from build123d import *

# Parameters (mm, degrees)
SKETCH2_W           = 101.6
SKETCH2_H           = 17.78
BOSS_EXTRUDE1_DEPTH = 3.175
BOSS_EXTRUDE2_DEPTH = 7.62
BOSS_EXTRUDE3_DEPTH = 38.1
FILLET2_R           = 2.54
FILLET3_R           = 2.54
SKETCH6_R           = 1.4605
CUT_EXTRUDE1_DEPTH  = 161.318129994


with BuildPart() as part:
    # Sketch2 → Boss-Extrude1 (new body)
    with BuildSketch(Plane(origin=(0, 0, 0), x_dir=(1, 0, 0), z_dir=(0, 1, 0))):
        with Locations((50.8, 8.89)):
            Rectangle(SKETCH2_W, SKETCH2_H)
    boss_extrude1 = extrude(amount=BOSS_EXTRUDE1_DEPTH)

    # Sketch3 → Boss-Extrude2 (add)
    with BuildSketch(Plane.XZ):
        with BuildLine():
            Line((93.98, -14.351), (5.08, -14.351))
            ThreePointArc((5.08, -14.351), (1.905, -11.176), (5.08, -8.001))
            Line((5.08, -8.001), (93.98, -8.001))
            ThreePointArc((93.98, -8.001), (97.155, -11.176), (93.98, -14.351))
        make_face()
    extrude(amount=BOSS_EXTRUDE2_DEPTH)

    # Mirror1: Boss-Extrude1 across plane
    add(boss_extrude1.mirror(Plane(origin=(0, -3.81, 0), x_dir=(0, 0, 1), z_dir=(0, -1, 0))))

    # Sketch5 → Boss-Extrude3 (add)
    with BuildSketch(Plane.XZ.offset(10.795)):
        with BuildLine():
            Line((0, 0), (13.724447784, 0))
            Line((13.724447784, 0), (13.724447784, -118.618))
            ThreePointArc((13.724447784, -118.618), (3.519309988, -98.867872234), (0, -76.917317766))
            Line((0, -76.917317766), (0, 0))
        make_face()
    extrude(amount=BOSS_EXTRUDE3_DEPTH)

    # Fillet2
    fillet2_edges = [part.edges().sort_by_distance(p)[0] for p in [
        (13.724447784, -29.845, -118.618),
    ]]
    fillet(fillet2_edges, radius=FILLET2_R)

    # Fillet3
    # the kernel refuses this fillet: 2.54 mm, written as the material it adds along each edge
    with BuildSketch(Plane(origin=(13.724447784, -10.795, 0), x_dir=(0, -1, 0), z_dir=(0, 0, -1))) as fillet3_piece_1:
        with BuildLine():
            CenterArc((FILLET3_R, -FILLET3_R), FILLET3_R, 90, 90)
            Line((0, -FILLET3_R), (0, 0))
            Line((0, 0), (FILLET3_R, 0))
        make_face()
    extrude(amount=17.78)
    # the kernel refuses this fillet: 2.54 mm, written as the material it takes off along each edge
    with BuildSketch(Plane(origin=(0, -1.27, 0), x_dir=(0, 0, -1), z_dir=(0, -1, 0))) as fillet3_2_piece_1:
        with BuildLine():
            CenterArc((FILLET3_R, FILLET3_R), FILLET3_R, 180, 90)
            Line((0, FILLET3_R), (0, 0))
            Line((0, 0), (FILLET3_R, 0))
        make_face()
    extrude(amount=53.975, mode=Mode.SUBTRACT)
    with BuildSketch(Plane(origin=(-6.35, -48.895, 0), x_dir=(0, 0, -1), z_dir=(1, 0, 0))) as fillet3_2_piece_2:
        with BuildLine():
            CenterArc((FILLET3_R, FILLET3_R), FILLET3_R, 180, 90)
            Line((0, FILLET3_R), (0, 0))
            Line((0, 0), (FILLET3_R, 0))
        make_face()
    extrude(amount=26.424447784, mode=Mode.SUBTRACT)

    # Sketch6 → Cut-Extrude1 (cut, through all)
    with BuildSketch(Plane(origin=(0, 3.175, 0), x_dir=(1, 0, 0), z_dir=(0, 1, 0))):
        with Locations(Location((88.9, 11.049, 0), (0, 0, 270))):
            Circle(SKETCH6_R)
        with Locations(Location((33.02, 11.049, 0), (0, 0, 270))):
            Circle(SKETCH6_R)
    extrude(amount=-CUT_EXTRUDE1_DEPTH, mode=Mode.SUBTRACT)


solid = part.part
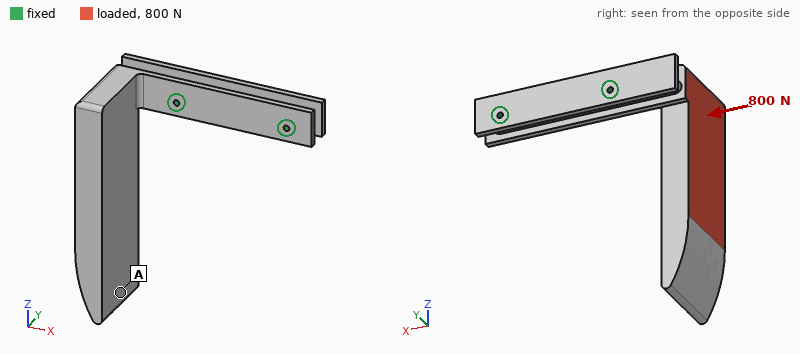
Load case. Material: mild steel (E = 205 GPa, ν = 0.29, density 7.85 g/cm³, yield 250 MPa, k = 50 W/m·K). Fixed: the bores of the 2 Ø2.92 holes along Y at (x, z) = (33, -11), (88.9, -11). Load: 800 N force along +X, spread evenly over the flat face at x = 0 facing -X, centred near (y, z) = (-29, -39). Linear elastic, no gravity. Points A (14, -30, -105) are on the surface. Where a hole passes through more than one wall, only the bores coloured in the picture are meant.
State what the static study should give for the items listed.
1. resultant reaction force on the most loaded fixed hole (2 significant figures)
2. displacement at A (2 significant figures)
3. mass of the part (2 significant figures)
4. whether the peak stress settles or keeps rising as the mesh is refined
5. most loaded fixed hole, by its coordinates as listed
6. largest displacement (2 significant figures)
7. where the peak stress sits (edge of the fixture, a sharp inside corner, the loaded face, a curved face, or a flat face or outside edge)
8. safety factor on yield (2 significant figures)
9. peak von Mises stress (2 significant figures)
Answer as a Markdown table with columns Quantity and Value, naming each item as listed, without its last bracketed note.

| Quantity | Value |
|---|---|
| resultant reaction force on the most loaded fixed hole | 1.2 kN |
| displacement at A | 0.22 mm |
| mass of the part | 550 g |
| whether the peak stress settles or keeps rising as the mesh is refined | settles |
| most loaded fixed hole, by its coordinates as listed | (33, -11) |
| largest displacement | 0.26 mm |
| where the peak stress sits | a curved face |
| safety factor on yield | 0.77 |
| peak von Mises stress | 320 MPa |
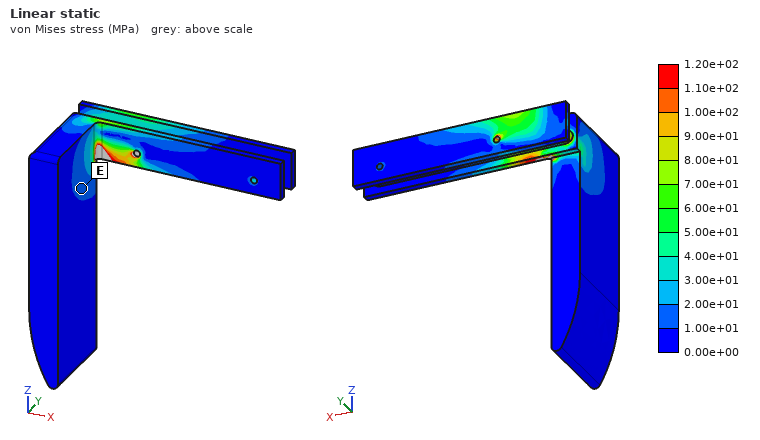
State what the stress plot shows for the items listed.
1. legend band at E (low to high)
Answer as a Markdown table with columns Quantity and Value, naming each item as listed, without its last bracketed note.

| Quantity | Value |
|---|---|
| legend band at E | 1.00e+01 to 2.00e+01 MPa |
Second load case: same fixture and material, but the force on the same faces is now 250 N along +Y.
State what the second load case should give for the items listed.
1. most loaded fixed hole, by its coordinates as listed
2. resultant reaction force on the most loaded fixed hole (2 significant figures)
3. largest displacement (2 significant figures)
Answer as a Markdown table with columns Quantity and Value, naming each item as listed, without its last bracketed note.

| Quantity | Value |
|---|---|
| most loaded fixed hole, by its coordinates as listed | (33, -11) |
| resultant reaction force on the most loaded fixed hole | 290 N |
| largest displacement | 0.16 mm |
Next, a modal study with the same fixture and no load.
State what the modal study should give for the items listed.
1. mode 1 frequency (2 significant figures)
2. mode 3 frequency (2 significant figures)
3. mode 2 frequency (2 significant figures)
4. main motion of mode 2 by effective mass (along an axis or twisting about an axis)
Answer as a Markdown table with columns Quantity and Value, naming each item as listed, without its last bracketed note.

| Quantity | Value |
|---|---|
| mode 1 frequency | 290 Hz |
| mode 3 frequency | 1500 Hz |
| mode 2 frequency | 470 Hz |
| main motion of mode 2 by effective mass | along X |
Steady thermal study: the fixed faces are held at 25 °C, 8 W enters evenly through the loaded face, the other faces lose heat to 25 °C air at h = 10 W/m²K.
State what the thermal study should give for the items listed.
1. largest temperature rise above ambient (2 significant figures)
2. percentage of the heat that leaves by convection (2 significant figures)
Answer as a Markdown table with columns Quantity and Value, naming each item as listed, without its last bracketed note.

| Quantity | Value |
|---|---|
| largest temperature rise above ambient | 28 K |
| percentage of the heat that leaves by convection | 33 % |
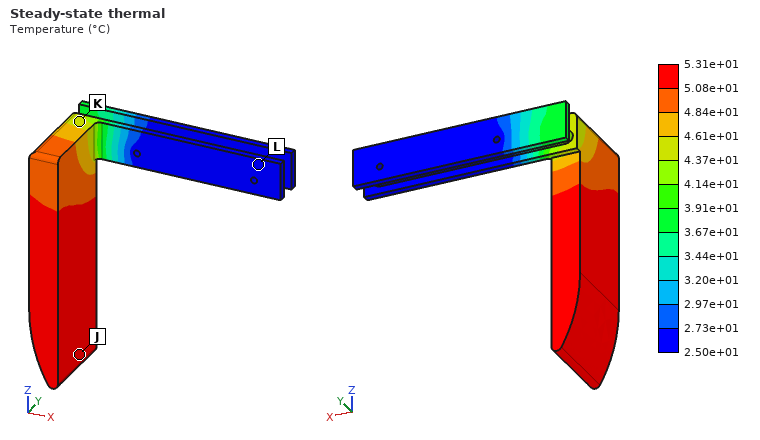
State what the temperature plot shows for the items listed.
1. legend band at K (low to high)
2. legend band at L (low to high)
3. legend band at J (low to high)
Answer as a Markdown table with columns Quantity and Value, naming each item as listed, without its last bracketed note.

| Quantity | Value |
|---|---|
| legend band at K | 4.37e+01 to 4.61e+01 °C |
| legend band at L | 2.50e+01 to 2.73e+01 °C |
| legend band at J | 5.08e+01 to 5.31e+01 °C |
